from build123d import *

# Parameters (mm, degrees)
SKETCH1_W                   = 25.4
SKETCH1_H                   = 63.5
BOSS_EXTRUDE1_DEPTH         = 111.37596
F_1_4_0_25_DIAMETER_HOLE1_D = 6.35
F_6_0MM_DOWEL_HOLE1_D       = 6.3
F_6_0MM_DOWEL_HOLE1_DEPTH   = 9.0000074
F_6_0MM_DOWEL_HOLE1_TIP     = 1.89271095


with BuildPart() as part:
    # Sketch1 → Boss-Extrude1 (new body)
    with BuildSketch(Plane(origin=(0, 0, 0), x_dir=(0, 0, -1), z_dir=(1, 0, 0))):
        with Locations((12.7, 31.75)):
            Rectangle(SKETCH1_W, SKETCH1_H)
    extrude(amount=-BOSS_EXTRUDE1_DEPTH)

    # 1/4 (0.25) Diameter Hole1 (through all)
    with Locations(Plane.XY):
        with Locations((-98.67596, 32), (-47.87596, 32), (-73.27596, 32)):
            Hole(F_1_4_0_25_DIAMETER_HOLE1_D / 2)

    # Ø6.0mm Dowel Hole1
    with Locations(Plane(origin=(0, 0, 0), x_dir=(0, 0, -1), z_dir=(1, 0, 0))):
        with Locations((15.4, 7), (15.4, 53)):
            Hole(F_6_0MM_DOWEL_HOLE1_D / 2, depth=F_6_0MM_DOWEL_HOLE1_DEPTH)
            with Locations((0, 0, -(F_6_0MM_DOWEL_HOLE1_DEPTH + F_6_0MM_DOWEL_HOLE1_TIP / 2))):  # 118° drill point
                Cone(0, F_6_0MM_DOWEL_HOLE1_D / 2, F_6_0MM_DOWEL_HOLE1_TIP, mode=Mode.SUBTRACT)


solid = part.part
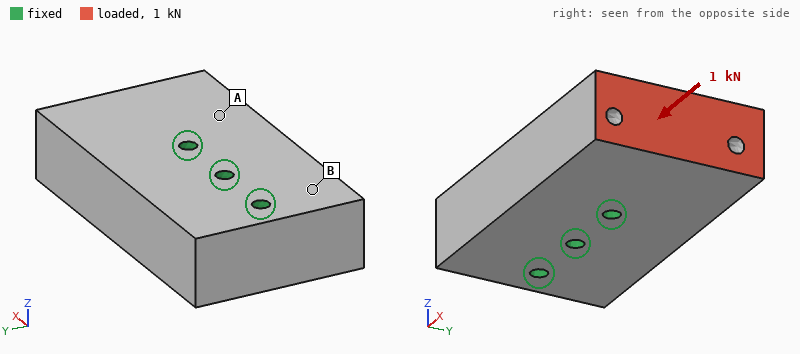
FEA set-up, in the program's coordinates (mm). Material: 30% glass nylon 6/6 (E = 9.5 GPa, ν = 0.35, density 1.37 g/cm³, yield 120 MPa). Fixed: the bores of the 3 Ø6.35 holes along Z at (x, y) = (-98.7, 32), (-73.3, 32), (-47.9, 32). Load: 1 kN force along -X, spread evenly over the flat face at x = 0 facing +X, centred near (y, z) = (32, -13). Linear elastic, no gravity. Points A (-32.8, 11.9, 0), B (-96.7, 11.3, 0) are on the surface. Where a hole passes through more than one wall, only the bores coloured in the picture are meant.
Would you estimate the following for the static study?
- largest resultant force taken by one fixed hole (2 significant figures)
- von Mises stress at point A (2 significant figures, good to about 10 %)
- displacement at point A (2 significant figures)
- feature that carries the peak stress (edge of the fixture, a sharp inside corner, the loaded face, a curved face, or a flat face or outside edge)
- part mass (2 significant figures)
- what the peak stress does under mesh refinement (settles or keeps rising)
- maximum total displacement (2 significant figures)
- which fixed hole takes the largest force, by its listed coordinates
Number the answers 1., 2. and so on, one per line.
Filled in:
1. 650 N
2. 0.53 MPa
3. 2.5 µm
4. edge of the fixture
5. 240 g
6. keeps rising
7. 4.7 µm
8. (-47.9, 32)
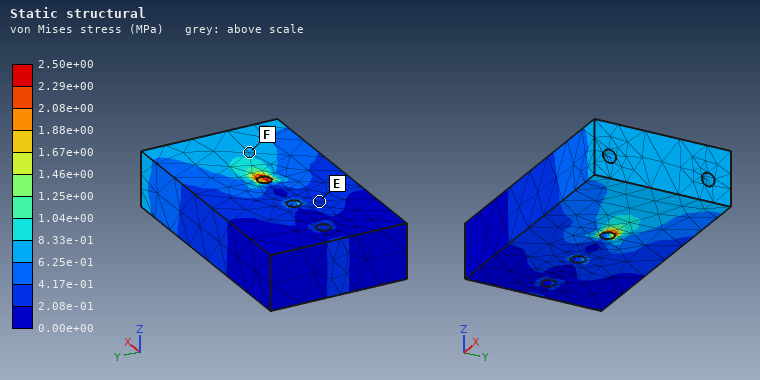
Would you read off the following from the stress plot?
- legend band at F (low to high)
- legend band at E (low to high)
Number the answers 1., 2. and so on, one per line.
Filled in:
1. 6.25e-01 to 8.33e-01 MPa
2. 2.08e-01 to 4.17e-01 MPa
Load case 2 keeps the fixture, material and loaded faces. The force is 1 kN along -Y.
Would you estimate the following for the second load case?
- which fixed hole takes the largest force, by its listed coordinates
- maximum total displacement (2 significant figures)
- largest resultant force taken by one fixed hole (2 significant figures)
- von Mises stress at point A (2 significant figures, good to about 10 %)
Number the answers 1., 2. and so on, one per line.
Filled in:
1. (-47.9, 32)
2. 43 µm
3. 1.9 kN
4. 1.6 MPa
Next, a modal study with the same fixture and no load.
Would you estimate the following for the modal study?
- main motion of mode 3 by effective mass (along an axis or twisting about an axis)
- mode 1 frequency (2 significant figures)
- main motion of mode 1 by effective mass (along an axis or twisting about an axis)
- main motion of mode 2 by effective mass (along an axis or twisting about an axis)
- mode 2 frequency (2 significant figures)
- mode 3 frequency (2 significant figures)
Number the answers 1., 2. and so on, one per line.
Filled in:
1. twisting about X
2. 3100 Hz
3. along Z
4. along Y
5. 3900 Hz
6. 4300 Hz
